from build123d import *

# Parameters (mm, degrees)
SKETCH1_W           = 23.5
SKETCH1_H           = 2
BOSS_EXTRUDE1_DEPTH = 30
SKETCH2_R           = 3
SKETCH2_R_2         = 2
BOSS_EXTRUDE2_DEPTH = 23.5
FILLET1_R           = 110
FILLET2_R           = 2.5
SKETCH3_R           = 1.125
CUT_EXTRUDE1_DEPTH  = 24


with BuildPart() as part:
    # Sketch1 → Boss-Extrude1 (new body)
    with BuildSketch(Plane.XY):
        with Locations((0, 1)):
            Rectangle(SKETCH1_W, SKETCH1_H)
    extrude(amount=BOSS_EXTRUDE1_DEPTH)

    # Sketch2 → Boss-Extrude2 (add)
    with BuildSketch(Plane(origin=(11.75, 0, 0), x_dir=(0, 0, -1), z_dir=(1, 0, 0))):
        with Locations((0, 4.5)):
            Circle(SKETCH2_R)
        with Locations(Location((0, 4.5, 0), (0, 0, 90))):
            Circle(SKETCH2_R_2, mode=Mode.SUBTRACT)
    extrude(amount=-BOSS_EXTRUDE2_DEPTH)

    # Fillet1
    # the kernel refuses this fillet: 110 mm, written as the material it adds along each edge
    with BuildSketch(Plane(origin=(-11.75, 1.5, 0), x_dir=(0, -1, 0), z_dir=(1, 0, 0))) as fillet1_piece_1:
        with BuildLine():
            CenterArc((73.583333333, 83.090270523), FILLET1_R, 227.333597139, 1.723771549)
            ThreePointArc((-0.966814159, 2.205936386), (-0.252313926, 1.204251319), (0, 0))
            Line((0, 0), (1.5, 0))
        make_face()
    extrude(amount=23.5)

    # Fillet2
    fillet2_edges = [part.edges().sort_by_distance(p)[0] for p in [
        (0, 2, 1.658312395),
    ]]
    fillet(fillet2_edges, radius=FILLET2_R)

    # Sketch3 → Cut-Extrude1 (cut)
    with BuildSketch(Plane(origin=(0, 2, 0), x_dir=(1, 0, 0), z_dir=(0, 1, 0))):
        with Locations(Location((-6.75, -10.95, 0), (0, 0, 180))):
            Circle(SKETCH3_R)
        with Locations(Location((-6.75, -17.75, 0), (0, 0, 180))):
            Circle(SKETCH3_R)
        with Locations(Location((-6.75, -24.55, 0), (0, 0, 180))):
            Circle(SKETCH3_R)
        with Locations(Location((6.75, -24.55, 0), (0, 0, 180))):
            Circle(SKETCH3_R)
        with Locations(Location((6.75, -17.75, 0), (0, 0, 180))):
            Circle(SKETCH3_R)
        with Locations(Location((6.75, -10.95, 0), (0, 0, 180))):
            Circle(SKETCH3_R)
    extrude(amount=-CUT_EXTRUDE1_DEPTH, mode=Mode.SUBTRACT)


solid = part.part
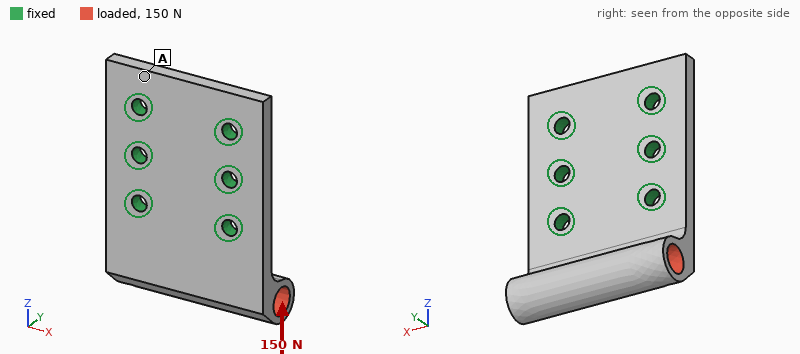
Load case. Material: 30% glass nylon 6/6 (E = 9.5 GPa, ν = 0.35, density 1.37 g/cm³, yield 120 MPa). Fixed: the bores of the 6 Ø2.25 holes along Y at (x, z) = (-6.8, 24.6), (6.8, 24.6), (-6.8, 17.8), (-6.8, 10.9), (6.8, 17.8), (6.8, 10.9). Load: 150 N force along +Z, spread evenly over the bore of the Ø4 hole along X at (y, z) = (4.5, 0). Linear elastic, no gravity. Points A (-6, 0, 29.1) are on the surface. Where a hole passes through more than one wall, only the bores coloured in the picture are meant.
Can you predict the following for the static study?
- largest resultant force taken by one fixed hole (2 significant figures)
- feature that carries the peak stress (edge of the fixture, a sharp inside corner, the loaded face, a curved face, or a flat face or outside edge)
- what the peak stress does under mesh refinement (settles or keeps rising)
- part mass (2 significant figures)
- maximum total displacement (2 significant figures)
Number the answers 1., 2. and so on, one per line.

1. 59 N
2. edge of the fixture
3. keeps rising
4. 2.5 g
5. 0.28 mm
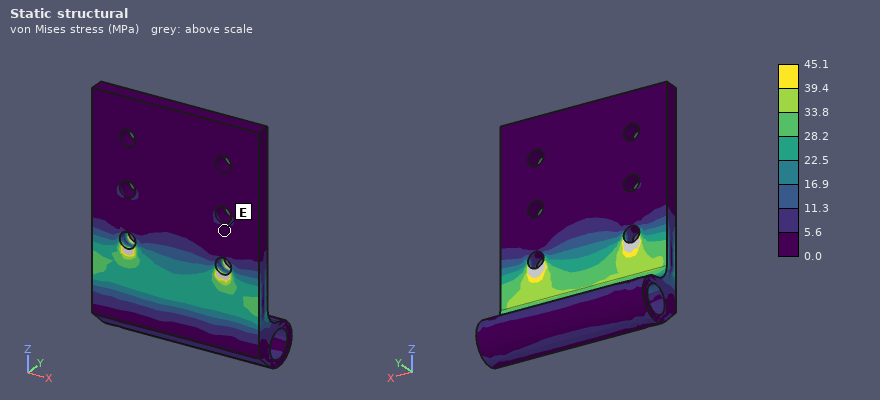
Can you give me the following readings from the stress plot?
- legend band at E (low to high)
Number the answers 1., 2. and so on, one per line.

1. 0.0 to 5.6 MPa
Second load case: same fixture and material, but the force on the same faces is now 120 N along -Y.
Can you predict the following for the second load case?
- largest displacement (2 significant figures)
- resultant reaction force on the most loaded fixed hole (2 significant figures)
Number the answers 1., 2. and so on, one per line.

1. 0.48 mm
2. 88 N
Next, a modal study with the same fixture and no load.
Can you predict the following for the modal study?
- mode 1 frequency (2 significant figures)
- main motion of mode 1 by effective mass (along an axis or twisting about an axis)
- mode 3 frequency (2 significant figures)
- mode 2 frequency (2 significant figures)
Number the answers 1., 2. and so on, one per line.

1. 3200 Hz
2. along Y
3. 16 kHz
4. 7600 Hz
